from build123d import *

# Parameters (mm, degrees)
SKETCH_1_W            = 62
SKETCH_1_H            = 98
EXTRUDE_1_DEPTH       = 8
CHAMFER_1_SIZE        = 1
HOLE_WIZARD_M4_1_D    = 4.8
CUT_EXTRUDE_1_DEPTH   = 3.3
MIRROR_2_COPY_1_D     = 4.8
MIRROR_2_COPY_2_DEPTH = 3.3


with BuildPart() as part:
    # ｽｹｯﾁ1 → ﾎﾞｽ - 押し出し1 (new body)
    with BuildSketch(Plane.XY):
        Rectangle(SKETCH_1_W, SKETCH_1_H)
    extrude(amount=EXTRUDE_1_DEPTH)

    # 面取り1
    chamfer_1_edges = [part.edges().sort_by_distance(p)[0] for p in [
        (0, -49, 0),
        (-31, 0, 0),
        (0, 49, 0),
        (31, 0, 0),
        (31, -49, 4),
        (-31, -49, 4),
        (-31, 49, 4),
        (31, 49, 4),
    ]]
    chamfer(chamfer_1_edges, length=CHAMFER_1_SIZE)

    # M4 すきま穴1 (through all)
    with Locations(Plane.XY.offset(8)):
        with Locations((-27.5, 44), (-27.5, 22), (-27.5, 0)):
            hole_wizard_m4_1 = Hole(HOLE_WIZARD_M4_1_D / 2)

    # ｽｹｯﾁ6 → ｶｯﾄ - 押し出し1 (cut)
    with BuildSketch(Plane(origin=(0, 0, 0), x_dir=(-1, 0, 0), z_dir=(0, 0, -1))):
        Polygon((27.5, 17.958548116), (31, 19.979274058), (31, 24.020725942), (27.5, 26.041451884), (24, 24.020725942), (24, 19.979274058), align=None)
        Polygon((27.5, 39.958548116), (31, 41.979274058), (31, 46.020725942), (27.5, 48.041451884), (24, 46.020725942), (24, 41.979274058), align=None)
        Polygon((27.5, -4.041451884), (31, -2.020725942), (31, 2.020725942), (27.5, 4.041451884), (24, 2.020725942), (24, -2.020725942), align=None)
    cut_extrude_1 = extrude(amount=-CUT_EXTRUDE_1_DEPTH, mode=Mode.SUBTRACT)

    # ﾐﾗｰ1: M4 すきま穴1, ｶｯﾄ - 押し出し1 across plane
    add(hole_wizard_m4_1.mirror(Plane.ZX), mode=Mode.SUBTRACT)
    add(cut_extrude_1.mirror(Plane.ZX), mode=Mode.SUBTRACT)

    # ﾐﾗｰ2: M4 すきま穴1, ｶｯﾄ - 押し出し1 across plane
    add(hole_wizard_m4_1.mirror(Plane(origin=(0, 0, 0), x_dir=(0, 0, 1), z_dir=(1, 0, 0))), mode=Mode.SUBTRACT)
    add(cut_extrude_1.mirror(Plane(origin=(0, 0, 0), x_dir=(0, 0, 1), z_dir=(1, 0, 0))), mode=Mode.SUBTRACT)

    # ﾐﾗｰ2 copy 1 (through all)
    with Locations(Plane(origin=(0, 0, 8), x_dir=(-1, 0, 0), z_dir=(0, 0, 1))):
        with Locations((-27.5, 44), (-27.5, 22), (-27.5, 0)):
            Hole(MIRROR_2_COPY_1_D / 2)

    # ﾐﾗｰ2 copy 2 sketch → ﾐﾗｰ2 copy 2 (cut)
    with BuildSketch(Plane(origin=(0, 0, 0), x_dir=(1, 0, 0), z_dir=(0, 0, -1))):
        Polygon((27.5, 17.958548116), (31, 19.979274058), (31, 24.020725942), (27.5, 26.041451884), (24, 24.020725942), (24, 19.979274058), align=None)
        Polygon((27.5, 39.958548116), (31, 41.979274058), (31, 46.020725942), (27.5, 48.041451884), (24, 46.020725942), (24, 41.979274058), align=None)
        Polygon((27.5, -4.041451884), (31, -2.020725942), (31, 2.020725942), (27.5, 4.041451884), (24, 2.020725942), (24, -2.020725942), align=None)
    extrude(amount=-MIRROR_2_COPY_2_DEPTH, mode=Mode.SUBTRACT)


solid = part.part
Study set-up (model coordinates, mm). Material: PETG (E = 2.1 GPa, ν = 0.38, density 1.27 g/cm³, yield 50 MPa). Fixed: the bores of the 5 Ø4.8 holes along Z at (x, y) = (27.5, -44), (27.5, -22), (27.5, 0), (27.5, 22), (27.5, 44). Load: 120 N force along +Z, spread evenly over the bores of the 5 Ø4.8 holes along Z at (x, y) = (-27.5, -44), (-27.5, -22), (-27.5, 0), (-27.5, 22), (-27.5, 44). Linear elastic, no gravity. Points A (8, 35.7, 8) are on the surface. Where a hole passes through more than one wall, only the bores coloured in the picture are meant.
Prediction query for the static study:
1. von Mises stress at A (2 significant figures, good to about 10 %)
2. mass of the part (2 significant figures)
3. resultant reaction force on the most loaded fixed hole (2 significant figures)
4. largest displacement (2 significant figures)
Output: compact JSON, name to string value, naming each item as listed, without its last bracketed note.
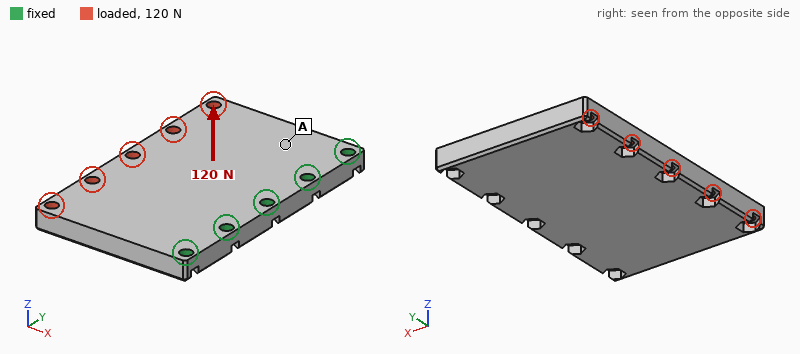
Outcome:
{"von Mises stress at A": "3.9 MPa", "mass of the part": "59 g", "resultant reaction force on the most loaded fixed hole": "42 N", "largest displacement": "1.3 mm"}
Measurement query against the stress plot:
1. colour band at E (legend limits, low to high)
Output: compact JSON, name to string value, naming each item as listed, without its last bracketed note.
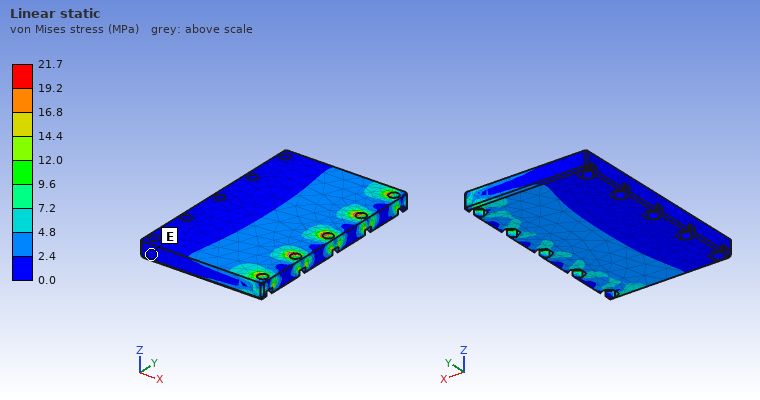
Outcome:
{"colour band at E": "0.0 to 2.4 MPa"}
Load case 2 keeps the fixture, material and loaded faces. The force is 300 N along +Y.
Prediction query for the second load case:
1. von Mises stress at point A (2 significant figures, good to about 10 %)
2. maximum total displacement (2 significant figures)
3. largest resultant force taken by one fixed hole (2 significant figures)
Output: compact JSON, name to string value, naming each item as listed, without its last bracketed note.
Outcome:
{"von Mises stress at point A": "1.2 MPa", "maximum total displacement": "0.14 mm", "largest resultant force taken by one fixed hole": "160 N"}
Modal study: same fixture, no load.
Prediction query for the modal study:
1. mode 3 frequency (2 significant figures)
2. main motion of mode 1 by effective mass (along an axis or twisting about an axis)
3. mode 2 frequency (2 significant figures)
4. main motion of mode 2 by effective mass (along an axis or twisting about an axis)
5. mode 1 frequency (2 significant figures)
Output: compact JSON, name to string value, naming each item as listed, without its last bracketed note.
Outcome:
{"mode 3 frequency": "1600 Hz", "main motion of mode 1 by effective mass": "along Z", "mode 2 frequency": "720 Hz", "main motion of mode 2 by effective mass": "twisting about X", "mode 1 frequency": "390 Hz"}
